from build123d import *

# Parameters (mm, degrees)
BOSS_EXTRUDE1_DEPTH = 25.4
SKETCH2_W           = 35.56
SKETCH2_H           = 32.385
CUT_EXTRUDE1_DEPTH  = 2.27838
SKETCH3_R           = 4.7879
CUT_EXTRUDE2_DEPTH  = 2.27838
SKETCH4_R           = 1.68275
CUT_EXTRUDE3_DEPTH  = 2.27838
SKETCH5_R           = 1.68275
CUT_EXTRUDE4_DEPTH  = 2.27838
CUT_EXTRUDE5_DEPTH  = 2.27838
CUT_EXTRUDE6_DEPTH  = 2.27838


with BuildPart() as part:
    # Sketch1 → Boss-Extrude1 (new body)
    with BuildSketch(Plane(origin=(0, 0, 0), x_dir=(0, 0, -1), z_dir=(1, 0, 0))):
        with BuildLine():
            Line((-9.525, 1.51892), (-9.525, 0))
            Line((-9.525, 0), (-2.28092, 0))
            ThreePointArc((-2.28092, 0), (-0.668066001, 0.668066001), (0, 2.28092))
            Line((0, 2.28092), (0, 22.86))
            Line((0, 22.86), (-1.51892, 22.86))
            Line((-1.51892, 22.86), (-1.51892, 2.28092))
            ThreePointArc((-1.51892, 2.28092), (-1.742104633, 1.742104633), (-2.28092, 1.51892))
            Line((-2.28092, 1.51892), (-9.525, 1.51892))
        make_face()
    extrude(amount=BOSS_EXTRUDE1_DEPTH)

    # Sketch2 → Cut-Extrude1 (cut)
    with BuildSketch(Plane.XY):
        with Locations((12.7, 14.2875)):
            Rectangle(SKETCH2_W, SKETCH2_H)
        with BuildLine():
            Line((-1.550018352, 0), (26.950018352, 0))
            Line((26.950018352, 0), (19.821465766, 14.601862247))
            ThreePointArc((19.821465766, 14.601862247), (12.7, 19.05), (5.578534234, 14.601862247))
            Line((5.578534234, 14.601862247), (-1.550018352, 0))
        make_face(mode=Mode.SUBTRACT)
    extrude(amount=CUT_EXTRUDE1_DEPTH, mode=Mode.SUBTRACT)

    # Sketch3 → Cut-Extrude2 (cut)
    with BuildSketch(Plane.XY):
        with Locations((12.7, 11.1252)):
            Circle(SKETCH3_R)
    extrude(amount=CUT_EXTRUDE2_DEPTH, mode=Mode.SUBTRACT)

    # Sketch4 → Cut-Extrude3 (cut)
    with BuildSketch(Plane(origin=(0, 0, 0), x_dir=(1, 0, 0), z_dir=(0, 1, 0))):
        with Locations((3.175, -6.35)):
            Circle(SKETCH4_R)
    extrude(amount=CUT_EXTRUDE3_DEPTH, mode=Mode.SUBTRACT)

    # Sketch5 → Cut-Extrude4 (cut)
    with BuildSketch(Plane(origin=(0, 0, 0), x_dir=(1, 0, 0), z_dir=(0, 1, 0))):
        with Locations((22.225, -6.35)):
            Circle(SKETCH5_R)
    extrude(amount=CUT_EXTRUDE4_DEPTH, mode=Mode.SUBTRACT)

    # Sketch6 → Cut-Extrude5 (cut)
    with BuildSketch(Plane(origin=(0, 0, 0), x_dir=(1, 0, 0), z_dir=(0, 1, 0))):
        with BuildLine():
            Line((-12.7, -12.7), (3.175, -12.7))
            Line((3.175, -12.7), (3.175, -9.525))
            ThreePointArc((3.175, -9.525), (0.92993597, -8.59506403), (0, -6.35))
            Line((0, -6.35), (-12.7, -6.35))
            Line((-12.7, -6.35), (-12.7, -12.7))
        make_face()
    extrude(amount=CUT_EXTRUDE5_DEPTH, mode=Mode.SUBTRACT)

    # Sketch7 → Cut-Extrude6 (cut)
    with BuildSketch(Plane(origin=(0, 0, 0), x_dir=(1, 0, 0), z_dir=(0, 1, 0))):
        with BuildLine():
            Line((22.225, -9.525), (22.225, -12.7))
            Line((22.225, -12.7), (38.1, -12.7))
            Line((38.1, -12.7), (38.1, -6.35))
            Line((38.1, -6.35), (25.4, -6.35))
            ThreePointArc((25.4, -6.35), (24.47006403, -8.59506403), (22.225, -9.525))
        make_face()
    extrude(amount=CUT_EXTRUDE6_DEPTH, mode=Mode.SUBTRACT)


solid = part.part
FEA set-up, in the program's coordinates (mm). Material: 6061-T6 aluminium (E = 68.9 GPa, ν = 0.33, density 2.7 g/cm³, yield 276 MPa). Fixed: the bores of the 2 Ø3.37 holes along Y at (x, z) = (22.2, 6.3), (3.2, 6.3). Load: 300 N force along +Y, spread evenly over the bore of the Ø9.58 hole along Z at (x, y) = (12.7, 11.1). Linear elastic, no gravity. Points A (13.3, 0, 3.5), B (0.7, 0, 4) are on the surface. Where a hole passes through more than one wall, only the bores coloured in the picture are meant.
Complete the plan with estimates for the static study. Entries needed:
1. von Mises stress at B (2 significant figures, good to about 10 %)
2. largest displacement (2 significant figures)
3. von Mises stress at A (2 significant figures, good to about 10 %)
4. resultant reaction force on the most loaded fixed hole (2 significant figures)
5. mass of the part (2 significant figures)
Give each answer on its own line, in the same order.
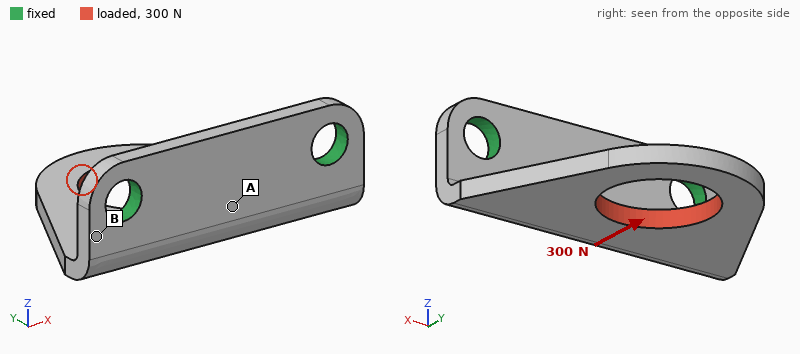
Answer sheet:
120 MPa
0.14 mm
31 MPa
150 N
1.8 g
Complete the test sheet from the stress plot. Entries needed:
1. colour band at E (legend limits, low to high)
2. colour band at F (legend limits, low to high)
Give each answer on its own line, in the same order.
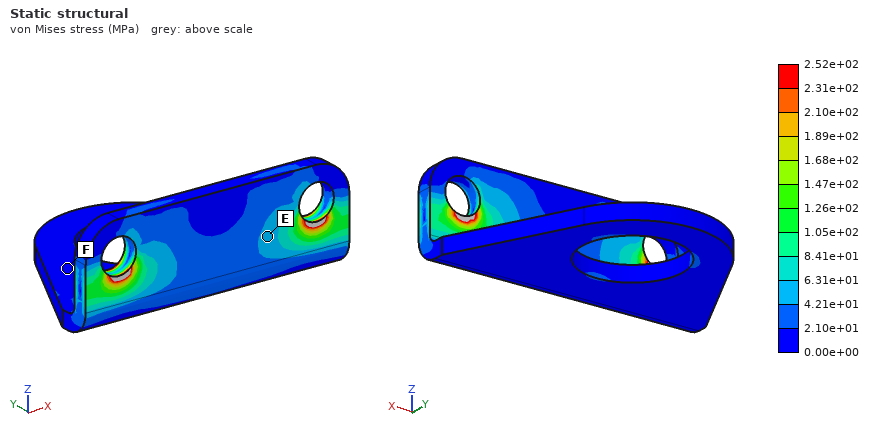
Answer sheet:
4.21e+01 to 6.31e+01 MPa
0.00e+00 to 2.10e+01 MPa
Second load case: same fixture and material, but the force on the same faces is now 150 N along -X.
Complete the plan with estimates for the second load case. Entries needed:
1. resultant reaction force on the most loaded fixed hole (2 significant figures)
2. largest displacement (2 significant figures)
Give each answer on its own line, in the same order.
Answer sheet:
110 N
30 µm
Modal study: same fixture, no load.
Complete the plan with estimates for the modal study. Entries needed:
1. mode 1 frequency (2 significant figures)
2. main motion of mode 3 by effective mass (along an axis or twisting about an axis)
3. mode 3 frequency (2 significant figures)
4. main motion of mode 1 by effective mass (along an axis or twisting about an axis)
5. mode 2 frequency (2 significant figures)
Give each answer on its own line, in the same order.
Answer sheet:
4100 Hz
along Y
15 kHz
along Z
10 kHz
